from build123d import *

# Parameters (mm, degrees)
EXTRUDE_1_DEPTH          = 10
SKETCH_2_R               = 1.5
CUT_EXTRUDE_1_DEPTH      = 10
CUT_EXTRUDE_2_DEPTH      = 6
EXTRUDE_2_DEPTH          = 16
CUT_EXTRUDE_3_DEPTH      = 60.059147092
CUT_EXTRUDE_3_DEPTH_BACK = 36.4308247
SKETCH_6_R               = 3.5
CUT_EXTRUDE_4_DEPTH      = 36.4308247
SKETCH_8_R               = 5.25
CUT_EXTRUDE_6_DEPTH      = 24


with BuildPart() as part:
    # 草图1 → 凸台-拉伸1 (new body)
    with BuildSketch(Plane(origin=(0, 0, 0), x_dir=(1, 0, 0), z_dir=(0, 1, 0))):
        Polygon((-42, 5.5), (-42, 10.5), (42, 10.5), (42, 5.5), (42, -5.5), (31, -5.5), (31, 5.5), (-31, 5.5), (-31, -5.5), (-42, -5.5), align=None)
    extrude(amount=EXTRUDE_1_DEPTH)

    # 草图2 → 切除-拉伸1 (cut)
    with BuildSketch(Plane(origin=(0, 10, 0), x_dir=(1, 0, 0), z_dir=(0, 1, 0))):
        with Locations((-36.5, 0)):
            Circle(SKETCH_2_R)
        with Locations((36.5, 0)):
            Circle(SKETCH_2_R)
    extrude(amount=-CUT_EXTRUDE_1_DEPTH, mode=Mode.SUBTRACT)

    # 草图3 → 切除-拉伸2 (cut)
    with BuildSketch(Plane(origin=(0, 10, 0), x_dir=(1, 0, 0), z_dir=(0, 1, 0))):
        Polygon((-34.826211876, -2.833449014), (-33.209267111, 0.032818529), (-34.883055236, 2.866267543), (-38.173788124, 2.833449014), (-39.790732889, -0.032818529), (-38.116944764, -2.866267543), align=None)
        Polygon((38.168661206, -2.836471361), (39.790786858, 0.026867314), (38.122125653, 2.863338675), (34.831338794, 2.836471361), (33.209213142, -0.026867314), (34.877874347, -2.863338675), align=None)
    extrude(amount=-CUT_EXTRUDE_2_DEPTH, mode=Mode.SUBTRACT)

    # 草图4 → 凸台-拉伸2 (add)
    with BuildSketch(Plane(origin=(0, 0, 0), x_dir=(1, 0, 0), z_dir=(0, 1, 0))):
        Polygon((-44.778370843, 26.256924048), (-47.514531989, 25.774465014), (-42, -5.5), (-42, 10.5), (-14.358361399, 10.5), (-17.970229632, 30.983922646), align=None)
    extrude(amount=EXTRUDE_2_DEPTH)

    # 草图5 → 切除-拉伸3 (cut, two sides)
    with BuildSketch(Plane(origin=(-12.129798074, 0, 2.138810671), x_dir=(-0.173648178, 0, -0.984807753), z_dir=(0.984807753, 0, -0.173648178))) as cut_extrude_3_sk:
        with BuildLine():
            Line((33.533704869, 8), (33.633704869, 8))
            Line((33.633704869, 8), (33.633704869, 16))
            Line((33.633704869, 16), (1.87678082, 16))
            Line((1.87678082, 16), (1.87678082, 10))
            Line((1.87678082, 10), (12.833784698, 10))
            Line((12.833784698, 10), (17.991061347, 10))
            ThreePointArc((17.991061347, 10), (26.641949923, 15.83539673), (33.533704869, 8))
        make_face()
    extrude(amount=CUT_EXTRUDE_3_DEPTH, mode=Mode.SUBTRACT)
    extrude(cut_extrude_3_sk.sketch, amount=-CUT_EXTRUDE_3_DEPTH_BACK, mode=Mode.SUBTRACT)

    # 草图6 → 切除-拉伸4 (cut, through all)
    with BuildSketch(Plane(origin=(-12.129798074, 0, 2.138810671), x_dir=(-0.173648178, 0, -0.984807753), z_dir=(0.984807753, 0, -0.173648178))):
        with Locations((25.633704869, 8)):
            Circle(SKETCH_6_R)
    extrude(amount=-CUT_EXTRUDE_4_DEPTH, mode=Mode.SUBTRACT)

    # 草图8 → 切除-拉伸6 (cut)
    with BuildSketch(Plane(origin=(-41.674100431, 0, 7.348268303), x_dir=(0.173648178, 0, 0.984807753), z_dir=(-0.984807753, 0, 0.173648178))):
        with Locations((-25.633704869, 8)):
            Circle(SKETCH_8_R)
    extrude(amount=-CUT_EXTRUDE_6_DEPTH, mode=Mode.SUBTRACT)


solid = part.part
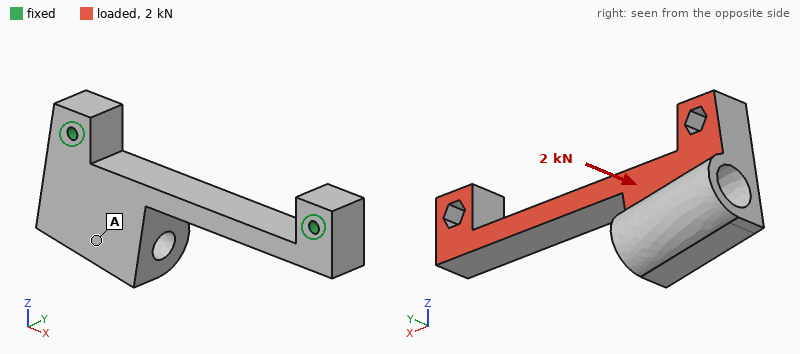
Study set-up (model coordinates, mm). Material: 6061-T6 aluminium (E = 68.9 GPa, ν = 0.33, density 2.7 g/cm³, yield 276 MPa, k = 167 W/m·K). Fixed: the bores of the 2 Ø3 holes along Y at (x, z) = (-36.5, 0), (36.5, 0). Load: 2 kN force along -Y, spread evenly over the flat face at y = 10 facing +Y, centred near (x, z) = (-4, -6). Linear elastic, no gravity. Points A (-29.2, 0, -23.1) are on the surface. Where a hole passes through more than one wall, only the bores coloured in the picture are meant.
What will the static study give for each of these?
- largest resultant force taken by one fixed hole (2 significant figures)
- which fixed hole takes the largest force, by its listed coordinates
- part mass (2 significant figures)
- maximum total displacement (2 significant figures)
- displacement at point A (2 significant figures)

1.1 kN
(-36.5, 0)
31 g
0.14 mm
0.091 mm
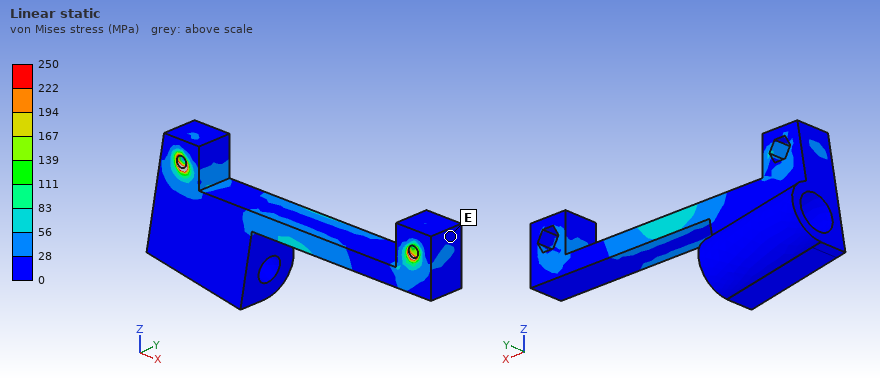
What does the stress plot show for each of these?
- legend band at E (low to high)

0 to 28 MPa
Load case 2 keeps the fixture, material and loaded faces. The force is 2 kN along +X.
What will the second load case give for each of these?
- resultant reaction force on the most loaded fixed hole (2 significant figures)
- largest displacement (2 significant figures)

1.0 kN
55 µm
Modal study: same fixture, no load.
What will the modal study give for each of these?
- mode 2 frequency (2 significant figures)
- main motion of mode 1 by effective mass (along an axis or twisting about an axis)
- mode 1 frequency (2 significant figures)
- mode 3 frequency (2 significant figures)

3900 Hz
along Y
2900 Hz
5800 Hz
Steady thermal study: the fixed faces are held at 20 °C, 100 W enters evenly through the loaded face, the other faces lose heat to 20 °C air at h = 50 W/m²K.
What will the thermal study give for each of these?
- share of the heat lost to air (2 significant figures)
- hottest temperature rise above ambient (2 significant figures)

9.5 %
63 K
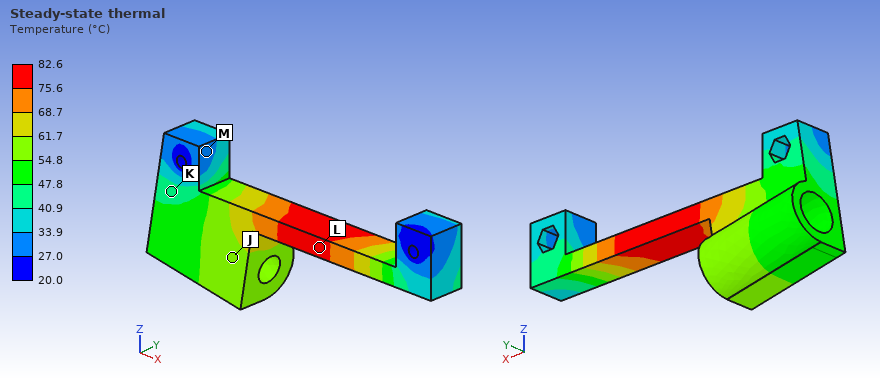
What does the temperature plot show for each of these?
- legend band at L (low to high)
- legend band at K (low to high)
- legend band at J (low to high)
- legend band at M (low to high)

75.6 to 82.6 °C
40.9 to 47.8 °C
54.8 to 61.7 °C
27.0 to 33.9 °C
